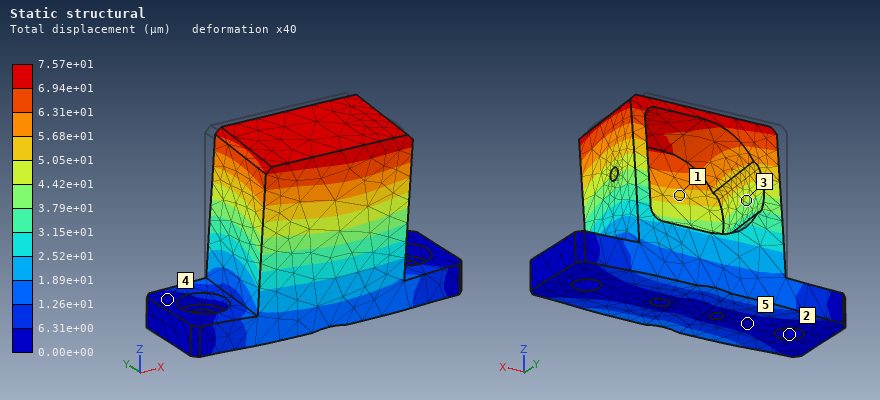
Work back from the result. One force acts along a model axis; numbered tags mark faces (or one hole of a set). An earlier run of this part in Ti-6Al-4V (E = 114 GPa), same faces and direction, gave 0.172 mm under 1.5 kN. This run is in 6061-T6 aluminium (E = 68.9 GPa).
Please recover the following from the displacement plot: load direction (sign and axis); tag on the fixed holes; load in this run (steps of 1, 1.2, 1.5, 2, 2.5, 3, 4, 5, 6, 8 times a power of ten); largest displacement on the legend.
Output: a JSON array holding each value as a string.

["-Y", "2", "400 N", "7.57e+01 µm"]
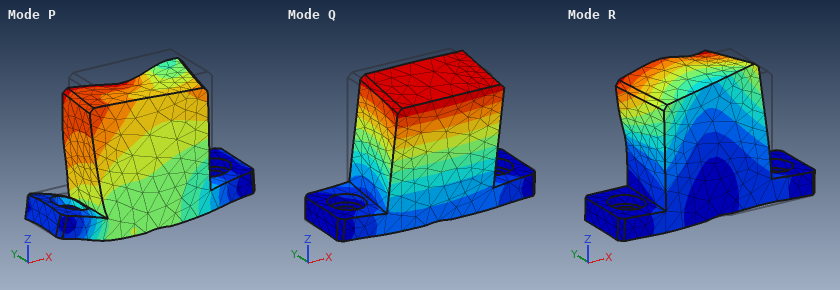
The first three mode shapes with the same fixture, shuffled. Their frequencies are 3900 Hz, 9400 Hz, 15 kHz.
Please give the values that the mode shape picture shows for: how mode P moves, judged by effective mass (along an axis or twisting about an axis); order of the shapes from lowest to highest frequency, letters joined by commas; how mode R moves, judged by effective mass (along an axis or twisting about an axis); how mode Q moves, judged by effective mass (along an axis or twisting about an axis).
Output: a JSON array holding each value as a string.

["along Z", "Q, R, P", "along X", "along Y"]
